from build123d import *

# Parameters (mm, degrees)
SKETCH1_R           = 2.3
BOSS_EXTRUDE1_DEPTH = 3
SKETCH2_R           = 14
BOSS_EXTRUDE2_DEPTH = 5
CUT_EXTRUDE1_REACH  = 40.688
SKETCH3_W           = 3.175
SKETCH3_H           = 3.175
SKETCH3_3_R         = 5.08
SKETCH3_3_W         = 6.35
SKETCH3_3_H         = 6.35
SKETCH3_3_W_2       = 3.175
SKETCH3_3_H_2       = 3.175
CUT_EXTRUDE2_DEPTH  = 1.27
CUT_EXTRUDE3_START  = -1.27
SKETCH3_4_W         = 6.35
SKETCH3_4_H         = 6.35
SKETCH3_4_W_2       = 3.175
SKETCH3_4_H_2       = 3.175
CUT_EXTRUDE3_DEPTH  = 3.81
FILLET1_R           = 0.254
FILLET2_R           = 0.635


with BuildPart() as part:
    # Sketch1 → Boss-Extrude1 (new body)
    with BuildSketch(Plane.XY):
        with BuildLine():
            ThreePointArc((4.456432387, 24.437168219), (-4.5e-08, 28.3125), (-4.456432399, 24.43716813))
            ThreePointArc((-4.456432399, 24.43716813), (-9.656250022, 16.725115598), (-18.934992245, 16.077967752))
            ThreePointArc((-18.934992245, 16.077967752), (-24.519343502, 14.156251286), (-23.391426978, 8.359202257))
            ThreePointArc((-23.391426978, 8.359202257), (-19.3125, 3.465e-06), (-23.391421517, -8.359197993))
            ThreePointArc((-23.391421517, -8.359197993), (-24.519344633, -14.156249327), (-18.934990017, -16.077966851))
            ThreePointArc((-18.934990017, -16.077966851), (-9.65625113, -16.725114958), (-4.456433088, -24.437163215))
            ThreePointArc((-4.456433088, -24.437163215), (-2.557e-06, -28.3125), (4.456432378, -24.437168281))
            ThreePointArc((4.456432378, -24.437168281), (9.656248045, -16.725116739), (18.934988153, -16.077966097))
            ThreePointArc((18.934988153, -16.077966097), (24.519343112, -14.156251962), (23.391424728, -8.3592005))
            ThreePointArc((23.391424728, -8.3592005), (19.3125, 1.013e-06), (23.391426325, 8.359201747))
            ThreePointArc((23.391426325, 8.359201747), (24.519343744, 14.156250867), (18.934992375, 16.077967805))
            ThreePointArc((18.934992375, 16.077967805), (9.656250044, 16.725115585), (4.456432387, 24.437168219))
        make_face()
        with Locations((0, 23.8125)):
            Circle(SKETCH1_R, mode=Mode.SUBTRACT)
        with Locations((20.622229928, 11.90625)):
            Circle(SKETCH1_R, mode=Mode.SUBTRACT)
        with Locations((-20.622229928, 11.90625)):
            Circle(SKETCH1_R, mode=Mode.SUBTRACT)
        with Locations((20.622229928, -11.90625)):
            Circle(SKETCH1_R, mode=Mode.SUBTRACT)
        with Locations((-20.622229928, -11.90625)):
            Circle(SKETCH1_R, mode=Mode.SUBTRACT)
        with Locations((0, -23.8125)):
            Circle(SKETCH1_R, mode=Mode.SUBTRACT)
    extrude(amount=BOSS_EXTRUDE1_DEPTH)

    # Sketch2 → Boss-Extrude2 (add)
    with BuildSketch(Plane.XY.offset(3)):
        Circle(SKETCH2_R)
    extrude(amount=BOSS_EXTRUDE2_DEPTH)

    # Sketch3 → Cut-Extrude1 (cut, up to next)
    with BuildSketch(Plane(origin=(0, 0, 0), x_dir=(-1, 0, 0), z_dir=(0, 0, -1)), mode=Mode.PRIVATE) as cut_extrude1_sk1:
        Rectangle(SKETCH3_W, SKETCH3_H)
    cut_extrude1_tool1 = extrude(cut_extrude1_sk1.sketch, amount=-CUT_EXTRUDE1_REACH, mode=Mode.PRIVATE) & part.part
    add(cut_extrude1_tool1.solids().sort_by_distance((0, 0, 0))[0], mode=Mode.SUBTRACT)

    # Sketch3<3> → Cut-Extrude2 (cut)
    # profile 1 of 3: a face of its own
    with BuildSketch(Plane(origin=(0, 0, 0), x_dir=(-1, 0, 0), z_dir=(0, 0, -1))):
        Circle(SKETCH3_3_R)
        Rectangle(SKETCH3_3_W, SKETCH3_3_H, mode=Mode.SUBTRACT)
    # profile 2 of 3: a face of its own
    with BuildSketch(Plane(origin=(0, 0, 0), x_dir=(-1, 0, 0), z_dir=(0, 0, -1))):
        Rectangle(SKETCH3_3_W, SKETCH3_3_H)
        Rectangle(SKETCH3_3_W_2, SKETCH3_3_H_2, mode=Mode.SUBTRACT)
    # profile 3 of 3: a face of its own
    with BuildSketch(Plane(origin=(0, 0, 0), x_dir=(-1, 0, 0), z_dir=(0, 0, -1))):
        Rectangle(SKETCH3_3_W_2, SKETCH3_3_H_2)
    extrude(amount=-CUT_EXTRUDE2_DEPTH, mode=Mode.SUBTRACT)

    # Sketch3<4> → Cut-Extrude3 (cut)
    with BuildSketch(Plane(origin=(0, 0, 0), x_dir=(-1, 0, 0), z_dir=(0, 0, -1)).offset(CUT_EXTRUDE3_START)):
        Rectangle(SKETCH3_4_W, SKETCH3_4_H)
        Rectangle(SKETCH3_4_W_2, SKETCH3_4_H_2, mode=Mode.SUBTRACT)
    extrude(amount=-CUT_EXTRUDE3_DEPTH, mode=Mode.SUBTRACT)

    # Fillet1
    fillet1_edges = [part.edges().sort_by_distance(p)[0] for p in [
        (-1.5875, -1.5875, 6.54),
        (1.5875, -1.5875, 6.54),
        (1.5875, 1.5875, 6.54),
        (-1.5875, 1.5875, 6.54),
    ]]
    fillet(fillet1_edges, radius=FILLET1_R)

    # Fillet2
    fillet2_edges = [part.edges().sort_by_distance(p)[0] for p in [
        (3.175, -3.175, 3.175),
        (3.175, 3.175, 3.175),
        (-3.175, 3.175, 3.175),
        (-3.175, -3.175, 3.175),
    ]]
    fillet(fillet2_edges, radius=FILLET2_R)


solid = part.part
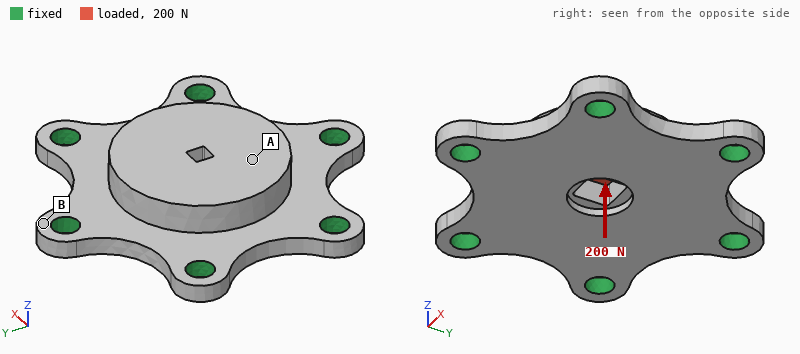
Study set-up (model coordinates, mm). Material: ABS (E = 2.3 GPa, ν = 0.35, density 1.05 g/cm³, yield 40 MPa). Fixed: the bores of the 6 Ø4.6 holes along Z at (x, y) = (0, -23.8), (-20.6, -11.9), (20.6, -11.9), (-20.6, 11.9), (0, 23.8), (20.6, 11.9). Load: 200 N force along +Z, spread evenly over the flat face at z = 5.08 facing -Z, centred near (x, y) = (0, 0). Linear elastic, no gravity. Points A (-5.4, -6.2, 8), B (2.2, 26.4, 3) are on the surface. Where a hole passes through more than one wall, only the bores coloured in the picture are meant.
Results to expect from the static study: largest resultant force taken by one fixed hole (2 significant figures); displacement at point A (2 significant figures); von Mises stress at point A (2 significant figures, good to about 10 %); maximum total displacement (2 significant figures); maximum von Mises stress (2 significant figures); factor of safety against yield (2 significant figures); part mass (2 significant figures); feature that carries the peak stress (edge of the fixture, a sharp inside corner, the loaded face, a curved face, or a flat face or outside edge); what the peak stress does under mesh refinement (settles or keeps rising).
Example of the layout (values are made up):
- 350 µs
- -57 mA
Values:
- 49 N
- 0.072 mm
- 2.6 MPa
- 0.11 mm
- 28 MPa
- 1.4
- 8.0 g
- a curved face
- settles
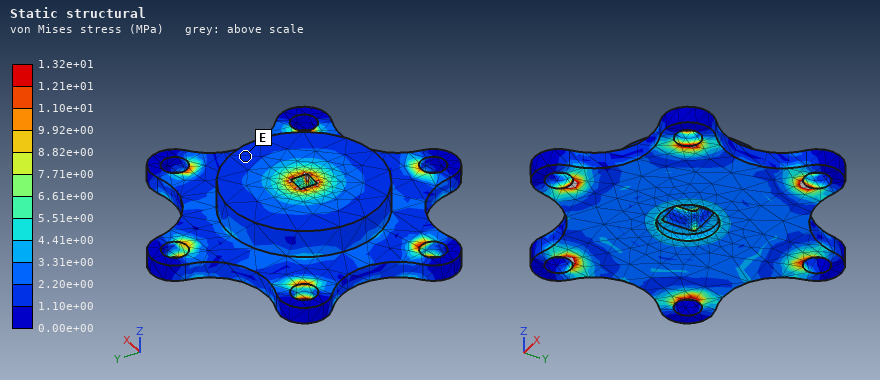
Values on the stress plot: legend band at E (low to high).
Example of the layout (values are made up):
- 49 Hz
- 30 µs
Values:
- 1.10e+00 to 2.20e+00 MPa
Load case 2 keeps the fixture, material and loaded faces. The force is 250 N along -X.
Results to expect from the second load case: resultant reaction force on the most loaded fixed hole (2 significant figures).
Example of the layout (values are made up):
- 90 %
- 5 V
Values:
- 62 N
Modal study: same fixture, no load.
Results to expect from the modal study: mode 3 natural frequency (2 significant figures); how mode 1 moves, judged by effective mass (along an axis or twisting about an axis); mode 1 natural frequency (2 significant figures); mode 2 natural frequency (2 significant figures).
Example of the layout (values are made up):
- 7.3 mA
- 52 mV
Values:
- 6300 Hz
- along Z
- 3900 Hz
- 6200 Hz
